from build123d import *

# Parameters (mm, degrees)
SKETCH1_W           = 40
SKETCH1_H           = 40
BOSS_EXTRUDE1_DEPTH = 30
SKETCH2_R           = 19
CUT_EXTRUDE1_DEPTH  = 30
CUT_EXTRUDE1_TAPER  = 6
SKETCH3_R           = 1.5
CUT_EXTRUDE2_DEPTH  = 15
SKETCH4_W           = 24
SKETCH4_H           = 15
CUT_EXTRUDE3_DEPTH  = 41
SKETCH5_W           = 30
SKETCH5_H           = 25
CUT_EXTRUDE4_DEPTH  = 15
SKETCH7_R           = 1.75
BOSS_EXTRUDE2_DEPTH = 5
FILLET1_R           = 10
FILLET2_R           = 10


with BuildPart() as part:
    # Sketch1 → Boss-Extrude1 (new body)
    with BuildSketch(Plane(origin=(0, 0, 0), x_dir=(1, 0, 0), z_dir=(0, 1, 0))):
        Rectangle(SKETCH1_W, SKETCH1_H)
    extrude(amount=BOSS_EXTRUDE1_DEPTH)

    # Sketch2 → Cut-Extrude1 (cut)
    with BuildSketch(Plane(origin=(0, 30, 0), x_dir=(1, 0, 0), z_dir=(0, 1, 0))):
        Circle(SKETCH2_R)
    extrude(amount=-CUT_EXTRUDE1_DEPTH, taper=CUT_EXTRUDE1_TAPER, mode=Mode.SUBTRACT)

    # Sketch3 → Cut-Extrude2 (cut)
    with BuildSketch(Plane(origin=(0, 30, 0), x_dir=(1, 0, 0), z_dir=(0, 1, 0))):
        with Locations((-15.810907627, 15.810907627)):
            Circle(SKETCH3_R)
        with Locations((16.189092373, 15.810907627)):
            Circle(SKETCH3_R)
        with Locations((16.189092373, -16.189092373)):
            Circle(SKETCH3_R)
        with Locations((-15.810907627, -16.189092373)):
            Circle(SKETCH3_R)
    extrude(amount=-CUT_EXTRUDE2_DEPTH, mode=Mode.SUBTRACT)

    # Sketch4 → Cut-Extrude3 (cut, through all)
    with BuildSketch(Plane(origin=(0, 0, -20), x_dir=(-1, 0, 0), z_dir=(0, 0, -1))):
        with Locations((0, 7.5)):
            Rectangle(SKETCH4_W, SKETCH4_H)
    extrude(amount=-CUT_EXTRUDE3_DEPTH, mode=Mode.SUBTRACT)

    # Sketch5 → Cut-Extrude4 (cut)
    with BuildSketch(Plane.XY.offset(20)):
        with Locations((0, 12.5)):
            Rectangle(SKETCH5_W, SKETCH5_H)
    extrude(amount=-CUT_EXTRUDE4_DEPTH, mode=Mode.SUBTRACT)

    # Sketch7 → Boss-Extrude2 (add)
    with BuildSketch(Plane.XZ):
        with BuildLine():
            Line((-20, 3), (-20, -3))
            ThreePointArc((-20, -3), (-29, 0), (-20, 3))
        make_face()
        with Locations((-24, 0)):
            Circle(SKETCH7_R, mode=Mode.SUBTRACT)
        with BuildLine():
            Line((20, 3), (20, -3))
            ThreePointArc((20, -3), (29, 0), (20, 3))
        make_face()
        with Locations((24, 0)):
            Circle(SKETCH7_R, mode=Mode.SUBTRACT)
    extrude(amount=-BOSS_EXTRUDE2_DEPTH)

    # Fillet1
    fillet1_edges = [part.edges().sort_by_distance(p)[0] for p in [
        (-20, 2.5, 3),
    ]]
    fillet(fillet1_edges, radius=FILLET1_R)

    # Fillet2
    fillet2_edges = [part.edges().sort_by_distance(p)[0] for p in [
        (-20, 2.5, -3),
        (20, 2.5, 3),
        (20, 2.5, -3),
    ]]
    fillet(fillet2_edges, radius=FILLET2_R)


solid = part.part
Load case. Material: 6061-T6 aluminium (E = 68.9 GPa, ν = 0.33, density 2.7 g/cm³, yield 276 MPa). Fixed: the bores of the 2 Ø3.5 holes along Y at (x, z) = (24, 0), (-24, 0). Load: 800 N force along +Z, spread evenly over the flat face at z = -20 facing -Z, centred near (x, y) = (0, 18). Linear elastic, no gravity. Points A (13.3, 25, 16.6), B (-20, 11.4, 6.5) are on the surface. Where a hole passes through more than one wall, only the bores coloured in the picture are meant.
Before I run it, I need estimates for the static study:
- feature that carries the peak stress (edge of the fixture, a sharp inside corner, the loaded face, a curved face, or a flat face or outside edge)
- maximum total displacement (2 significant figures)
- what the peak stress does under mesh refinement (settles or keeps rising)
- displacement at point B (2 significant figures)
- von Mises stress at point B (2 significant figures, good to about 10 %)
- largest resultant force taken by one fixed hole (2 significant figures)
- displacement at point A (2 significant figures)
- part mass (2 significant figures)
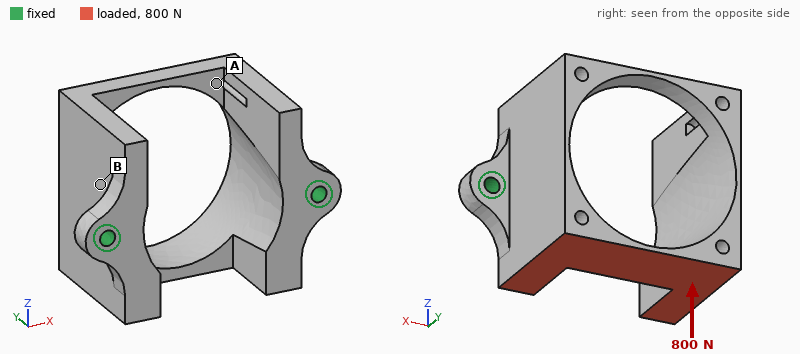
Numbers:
edge of the fixture
0.12 mm
keeps rising
0.031 mm
19 MPa
410 N
0.069 mm
38 g
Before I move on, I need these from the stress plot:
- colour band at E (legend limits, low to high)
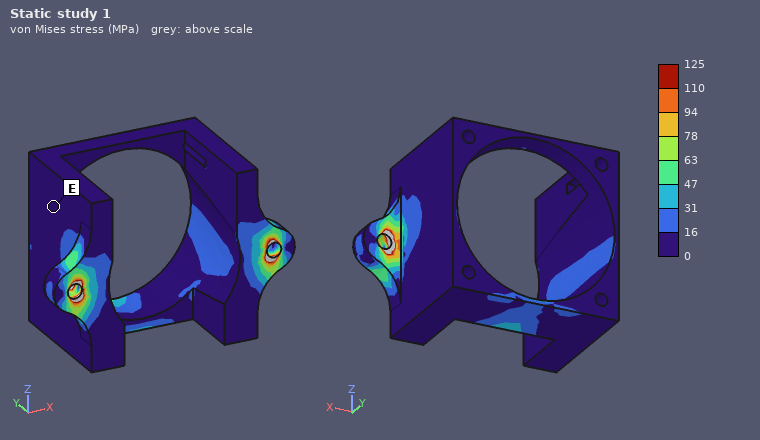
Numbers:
0 to 16 MPa
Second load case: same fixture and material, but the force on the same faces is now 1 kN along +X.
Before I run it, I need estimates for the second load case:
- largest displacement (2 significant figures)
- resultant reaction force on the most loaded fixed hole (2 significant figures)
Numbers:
55 µm
650 N
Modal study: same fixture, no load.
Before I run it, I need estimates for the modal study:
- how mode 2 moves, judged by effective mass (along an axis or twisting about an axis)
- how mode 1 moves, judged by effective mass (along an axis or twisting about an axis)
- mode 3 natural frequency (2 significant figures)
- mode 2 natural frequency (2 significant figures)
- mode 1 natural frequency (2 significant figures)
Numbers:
along X
along Z
5200 Hz
4000 Hz
2900 Hz
